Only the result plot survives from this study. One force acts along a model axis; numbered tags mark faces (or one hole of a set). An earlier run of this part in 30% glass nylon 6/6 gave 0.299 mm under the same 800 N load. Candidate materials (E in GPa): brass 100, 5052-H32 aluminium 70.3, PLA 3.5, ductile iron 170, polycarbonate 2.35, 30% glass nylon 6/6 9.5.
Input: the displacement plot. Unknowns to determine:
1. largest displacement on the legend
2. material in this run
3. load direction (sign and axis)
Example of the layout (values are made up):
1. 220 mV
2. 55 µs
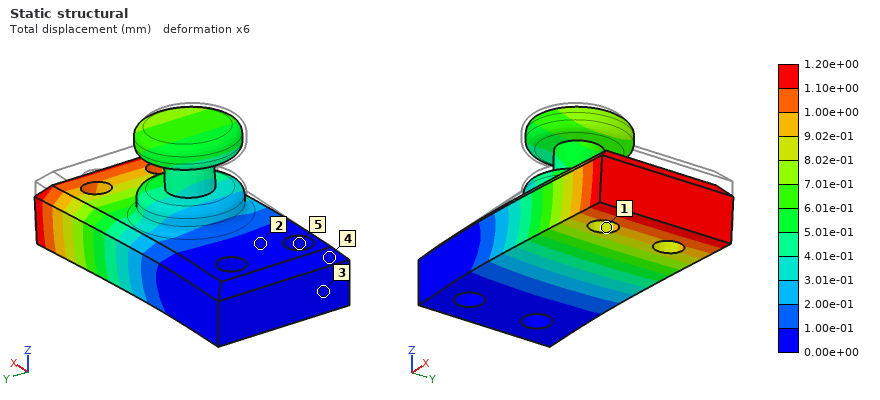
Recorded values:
1. 1.20e+00 mm
2. polycarbonate
3. -Z
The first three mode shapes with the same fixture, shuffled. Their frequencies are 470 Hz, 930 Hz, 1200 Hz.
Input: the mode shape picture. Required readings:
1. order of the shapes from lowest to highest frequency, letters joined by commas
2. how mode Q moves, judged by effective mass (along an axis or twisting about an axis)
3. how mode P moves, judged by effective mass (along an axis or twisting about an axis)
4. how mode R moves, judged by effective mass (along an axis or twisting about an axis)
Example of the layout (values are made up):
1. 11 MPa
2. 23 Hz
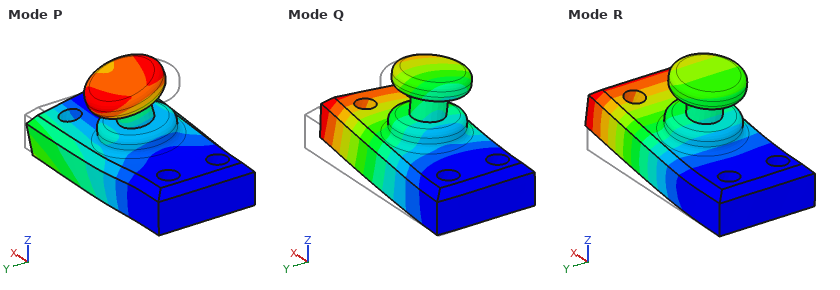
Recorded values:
1. R, Q, P
2. along Y
3. twisting about X
4. along Z
